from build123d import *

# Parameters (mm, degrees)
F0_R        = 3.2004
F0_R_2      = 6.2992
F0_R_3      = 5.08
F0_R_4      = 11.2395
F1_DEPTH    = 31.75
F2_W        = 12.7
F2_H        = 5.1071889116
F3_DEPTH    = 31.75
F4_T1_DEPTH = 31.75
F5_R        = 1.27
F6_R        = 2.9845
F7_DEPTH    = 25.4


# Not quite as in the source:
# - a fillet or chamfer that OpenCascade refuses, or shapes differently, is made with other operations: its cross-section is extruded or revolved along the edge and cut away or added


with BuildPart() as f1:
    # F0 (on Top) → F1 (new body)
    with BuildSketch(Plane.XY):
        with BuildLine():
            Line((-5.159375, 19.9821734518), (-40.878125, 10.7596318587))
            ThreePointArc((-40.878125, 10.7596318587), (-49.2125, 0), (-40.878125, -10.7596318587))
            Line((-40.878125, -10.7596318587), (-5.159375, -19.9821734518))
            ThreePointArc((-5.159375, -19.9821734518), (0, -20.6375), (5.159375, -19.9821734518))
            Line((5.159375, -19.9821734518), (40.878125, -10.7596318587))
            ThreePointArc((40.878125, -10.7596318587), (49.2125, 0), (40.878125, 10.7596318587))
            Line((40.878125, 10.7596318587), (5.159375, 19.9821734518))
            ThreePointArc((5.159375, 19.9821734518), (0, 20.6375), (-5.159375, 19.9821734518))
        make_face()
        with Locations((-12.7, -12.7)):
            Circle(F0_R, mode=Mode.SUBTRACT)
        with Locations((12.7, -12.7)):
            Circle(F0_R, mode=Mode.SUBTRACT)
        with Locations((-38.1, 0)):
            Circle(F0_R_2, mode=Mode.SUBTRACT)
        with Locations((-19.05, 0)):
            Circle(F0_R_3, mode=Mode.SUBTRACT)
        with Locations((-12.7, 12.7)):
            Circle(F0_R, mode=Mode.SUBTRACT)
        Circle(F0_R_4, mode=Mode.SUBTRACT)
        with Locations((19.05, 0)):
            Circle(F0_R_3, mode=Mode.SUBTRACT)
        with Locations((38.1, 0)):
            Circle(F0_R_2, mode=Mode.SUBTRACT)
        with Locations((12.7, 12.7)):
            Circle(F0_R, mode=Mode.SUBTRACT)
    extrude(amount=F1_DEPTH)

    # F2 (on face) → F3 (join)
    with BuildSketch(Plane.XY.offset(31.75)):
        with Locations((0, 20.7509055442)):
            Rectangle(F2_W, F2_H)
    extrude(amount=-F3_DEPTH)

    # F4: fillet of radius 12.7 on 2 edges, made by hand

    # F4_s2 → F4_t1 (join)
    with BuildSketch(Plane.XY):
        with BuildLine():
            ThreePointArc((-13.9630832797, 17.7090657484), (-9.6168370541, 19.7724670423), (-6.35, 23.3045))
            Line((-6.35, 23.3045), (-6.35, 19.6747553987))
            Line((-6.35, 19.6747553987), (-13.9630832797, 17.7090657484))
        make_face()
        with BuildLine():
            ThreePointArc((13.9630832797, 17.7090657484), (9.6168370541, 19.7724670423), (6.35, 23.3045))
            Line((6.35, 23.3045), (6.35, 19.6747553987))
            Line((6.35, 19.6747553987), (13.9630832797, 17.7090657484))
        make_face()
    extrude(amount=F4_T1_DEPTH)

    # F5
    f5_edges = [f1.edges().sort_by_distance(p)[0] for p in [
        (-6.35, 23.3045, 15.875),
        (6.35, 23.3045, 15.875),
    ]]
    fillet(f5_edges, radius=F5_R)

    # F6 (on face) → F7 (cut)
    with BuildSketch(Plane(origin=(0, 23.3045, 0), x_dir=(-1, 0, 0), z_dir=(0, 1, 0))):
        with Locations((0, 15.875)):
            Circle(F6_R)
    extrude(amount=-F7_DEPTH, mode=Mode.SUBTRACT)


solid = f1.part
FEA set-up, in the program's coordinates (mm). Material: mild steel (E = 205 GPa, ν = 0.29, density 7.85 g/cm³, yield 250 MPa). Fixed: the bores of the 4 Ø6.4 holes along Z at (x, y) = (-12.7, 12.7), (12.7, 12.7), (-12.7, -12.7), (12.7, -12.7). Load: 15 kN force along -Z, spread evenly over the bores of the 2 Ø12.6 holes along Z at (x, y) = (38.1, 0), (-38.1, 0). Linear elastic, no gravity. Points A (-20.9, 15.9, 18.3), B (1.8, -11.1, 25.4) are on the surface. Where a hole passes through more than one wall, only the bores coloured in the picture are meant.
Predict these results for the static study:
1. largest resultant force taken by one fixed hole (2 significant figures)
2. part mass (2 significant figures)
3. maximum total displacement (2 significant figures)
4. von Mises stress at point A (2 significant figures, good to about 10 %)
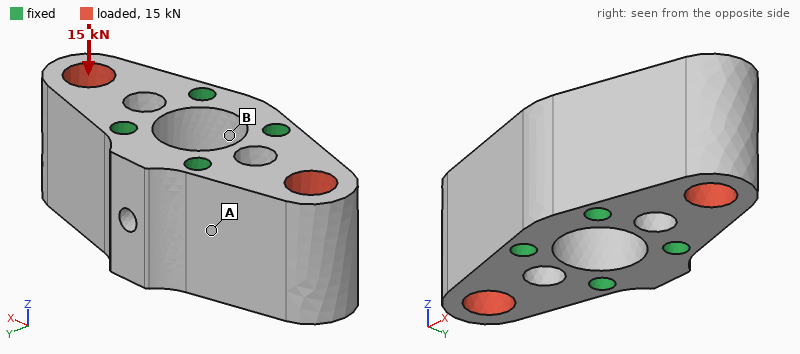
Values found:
3.8 kN
500 g
11 µm
24 MPa
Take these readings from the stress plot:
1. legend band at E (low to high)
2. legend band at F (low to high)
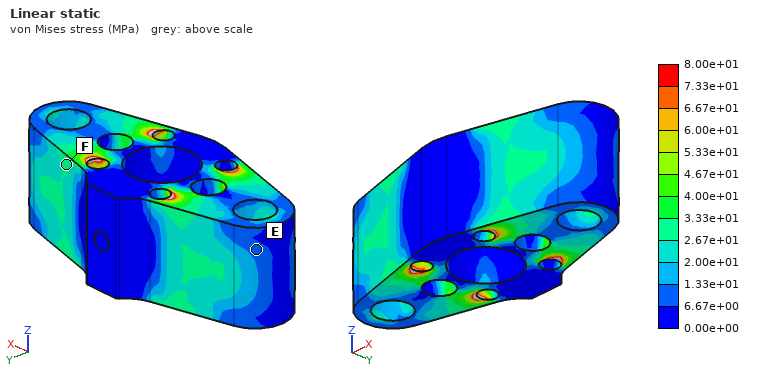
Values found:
6.67e+00 to 1.33e+01 MPa
2.67e+01 to 3.33e+01 MPa
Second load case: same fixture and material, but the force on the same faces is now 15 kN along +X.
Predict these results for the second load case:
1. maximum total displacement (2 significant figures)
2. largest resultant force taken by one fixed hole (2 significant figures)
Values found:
2.4 µm
3.9 kN
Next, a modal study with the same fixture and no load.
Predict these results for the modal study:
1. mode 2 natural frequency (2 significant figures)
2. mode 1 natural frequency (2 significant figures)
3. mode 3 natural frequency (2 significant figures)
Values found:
17 kHz
17 kHz
18 kHz
